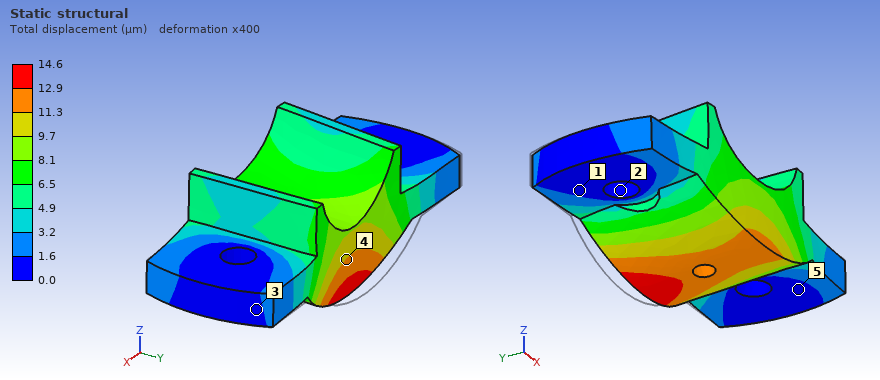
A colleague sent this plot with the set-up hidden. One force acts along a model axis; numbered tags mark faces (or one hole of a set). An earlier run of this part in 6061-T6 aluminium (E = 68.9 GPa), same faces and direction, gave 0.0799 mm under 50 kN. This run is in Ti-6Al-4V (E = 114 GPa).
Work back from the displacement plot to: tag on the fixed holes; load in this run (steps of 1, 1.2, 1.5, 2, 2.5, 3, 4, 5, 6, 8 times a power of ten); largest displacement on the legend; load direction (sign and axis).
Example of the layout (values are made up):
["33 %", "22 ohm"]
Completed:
["2", "15 kN", "14.6 µm", "-Y"]
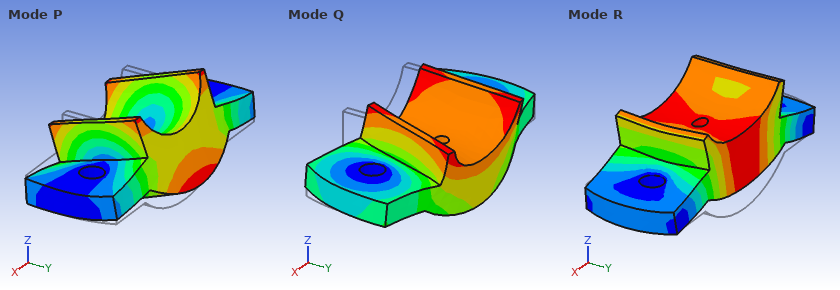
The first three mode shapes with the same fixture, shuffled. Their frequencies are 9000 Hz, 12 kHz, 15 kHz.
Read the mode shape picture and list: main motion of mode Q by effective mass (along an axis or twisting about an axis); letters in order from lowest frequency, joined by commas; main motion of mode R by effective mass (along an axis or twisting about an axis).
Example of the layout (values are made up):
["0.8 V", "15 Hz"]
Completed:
["along Y", "P, R, Q", "along Z"]
